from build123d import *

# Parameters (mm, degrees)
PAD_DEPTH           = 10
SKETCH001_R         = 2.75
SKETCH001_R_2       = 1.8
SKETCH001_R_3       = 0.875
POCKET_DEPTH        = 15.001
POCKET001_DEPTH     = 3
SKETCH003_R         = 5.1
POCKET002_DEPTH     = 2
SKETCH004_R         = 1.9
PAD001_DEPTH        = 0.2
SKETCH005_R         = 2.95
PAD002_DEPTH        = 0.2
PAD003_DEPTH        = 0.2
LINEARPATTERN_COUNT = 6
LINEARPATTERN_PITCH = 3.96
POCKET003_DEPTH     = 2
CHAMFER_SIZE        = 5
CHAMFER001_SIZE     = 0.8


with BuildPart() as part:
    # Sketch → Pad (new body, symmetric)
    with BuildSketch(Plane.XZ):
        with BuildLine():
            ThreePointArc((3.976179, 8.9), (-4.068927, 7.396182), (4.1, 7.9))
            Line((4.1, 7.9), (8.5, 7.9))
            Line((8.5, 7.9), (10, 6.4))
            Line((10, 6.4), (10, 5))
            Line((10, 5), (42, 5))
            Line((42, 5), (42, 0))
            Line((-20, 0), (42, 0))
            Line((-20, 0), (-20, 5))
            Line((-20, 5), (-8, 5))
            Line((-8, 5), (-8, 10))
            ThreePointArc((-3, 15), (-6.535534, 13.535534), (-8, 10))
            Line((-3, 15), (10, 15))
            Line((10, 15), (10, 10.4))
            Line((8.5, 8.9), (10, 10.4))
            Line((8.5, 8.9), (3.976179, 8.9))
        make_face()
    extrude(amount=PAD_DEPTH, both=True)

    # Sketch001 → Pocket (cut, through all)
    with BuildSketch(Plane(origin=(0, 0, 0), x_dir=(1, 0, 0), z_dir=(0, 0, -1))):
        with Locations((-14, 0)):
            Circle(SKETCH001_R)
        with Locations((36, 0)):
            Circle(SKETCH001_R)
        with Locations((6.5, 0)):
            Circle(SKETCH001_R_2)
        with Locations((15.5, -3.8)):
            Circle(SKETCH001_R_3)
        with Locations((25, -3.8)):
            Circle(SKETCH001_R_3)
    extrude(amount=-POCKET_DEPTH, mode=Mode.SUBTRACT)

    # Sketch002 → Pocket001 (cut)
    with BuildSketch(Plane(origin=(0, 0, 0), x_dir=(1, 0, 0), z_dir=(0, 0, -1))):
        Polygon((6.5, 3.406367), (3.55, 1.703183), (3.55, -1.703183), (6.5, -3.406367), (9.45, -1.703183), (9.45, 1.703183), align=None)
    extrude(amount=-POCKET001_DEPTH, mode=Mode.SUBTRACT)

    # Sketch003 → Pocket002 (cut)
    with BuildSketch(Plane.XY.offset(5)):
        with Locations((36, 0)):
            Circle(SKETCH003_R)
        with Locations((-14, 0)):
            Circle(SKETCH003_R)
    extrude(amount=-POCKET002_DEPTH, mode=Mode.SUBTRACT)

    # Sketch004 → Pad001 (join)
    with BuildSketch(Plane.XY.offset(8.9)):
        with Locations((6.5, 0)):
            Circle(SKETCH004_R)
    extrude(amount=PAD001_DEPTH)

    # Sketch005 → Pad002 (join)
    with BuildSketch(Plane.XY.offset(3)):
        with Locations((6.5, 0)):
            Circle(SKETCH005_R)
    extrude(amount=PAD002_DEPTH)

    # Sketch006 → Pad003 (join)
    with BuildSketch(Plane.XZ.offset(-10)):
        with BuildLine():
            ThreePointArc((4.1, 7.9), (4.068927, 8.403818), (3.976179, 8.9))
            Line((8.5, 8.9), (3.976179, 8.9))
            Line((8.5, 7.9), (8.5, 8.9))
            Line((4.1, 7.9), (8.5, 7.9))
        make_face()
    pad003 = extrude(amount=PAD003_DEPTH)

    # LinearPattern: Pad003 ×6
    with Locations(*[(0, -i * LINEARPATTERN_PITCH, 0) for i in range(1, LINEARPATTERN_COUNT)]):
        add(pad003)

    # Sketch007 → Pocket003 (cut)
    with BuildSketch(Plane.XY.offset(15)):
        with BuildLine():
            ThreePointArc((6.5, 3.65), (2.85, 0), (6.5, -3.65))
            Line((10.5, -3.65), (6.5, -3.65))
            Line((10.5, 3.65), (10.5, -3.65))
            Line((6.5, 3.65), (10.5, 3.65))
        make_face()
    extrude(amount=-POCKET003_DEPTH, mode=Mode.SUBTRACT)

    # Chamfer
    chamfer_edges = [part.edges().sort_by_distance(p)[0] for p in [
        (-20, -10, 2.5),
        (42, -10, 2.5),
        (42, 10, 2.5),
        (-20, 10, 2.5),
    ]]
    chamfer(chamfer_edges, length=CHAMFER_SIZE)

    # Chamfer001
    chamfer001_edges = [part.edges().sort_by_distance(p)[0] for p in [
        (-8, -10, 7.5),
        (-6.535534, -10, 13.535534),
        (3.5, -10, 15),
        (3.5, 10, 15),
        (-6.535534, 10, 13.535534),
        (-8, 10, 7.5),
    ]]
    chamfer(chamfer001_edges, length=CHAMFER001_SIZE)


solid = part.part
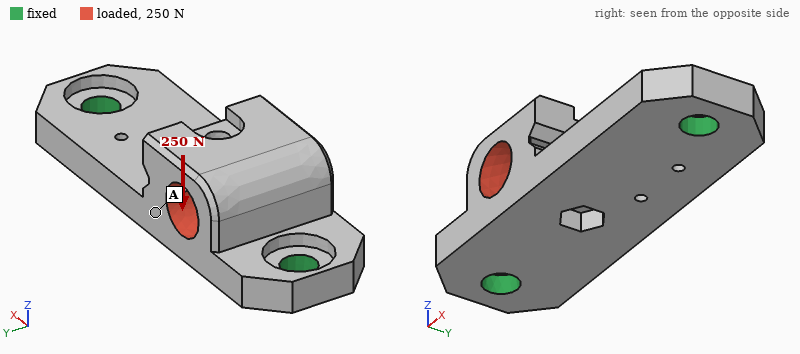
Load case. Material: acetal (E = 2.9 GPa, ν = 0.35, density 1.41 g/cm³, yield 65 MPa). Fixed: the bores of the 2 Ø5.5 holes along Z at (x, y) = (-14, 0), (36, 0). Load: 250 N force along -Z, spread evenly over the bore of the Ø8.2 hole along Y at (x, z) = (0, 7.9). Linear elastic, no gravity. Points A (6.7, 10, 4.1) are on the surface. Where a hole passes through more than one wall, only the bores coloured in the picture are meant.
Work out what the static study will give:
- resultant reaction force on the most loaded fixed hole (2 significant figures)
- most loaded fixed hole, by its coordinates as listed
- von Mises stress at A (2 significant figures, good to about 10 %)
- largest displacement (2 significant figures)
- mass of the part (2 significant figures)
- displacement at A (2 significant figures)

220 N
(-14, 0)
4.3 MPa
0.26 mm
11 g
0.20 mm
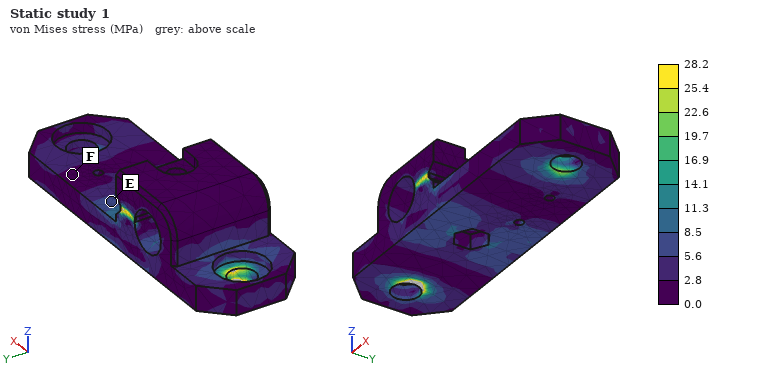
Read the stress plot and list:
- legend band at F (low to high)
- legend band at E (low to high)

0.0 to 2.8 MPa
5.6 to 8.5 MPa
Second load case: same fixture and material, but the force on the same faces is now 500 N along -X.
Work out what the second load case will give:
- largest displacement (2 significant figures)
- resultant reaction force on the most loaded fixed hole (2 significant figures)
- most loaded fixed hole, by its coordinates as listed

0.26 mm
280 N
(-14, 0)
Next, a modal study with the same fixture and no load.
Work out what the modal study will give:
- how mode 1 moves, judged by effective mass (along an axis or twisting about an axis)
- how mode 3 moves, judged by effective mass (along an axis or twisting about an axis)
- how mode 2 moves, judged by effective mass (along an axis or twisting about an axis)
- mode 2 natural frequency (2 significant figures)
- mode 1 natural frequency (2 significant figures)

along Z
along Y
along Y
2100 Hz
2000 Hz
